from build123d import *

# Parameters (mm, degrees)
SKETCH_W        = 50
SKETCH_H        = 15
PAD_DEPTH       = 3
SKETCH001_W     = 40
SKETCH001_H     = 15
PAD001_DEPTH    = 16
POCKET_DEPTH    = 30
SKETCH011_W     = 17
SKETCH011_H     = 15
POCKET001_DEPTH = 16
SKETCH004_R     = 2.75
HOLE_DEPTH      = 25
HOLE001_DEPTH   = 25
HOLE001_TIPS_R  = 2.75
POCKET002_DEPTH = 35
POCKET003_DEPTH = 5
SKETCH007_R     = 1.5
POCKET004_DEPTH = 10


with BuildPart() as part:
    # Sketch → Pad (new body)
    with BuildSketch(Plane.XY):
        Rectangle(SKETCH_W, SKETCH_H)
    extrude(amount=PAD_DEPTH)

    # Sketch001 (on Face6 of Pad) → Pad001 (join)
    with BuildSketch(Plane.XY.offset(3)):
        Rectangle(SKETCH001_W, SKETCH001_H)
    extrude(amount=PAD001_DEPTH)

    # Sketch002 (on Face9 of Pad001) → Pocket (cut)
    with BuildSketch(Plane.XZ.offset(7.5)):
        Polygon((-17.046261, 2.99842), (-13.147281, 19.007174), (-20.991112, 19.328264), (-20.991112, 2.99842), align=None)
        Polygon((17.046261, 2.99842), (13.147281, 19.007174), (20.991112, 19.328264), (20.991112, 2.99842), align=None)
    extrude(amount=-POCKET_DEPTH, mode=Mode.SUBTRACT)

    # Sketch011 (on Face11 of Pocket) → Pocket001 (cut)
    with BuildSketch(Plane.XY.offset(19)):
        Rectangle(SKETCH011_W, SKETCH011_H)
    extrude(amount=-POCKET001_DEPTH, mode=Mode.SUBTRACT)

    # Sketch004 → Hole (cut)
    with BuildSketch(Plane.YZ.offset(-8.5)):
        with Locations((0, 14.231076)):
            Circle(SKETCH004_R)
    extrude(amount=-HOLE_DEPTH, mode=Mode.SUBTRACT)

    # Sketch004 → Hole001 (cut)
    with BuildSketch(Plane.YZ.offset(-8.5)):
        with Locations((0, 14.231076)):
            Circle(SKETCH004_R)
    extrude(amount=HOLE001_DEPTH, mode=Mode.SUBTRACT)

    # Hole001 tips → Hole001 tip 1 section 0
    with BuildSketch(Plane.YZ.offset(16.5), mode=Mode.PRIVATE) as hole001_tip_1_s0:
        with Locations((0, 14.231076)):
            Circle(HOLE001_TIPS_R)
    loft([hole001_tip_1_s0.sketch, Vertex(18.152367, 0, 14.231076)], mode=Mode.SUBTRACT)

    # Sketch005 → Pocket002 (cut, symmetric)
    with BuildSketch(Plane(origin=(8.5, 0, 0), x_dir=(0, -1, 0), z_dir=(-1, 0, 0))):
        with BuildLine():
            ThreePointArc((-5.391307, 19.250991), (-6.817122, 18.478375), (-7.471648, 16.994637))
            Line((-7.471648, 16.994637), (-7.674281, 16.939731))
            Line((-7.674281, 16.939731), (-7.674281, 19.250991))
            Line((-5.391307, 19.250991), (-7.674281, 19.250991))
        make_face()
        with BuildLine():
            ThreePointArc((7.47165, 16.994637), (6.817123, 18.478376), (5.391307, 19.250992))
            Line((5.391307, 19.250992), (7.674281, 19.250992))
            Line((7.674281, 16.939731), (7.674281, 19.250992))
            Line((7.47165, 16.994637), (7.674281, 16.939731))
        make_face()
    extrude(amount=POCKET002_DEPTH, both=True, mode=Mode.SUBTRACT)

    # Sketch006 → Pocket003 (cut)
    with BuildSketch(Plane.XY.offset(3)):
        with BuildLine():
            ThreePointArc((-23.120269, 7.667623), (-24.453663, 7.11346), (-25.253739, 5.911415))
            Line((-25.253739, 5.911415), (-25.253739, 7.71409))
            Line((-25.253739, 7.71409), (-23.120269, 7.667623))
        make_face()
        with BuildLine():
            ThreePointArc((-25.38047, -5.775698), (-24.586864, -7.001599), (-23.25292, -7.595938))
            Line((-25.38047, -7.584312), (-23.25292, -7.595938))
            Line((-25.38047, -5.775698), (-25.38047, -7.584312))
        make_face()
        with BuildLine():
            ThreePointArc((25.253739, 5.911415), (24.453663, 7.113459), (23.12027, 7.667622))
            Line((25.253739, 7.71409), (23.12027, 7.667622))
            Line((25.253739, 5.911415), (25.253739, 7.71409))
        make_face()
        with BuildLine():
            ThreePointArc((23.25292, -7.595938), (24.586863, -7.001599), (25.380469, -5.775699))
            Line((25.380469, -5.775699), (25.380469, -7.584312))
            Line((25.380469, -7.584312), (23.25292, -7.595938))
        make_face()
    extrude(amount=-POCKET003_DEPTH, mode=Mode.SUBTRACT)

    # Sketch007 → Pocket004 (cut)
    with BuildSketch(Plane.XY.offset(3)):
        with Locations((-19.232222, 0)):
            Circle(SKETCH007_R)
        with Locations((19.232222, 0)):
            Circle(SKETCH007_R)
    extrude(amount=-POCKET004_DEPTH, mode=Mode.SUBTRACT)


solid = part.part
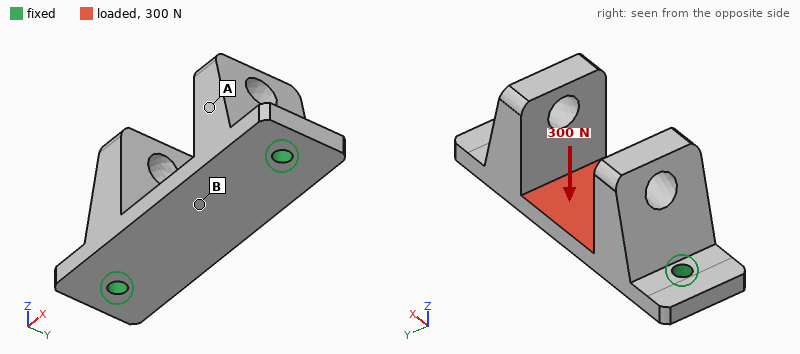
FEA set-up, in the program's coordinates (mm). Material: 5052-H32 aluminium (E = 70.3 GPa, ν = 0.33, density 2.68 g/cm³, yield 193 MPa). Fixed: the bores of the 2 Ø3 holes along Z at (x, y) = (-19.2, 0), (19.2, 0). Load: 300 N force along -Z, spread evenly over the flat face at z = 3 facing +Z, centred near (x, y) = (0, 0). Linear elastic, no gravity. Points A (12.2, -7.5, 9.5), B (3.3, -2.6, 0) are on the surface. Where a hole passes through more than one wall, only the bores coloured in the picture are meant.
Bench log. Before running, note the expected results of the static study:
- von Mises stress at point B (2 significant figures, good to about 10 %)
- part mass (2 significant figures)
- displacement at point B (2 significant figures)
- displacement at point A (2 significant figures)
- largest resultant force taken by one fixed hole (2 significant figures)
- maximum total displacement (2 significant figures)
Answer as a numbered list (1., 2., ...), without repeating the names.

1. 28 MPa
2. 14 g
3. 27 µm
4. 19 µm
5. 150 N
6. 39 µm
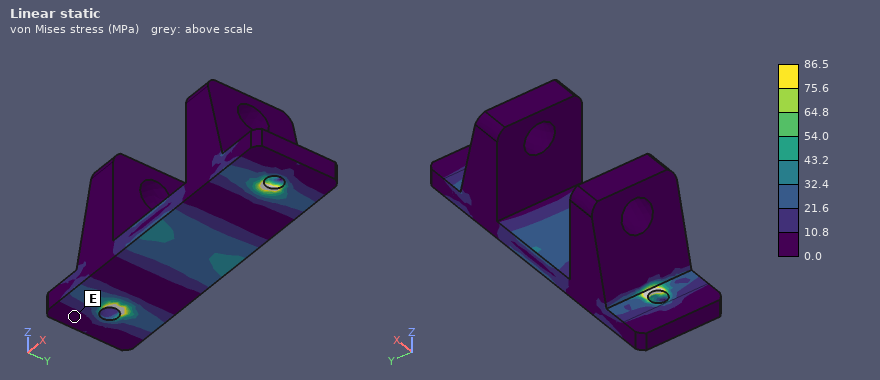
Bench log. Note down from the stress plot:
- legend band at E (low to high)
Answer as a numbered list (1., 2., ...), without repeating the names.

1. 0.0 to 10.8 MPa
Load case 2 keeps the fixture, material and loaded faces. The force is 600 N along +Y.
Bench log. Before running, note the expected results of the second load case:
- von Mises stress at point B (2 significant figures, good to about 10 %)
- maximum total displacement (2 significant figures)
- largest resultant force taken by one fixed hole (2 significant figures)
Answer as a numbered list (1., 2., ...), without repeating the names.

1. 10 MPa
2. 13 µm
3. 300 N
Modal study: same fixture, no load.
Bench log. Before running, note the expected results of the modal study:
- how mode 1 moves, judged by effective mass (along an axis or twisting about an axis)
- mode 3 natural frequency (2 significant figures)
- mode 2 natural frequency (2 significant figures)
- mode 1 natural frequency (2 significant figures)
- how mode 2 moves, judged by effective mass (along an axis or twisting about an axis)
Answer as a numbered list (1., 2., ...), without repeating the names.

1. along Z
2. 9200 Hz
3. 7600 Hz
4. 5700 Hz
5. along Y
